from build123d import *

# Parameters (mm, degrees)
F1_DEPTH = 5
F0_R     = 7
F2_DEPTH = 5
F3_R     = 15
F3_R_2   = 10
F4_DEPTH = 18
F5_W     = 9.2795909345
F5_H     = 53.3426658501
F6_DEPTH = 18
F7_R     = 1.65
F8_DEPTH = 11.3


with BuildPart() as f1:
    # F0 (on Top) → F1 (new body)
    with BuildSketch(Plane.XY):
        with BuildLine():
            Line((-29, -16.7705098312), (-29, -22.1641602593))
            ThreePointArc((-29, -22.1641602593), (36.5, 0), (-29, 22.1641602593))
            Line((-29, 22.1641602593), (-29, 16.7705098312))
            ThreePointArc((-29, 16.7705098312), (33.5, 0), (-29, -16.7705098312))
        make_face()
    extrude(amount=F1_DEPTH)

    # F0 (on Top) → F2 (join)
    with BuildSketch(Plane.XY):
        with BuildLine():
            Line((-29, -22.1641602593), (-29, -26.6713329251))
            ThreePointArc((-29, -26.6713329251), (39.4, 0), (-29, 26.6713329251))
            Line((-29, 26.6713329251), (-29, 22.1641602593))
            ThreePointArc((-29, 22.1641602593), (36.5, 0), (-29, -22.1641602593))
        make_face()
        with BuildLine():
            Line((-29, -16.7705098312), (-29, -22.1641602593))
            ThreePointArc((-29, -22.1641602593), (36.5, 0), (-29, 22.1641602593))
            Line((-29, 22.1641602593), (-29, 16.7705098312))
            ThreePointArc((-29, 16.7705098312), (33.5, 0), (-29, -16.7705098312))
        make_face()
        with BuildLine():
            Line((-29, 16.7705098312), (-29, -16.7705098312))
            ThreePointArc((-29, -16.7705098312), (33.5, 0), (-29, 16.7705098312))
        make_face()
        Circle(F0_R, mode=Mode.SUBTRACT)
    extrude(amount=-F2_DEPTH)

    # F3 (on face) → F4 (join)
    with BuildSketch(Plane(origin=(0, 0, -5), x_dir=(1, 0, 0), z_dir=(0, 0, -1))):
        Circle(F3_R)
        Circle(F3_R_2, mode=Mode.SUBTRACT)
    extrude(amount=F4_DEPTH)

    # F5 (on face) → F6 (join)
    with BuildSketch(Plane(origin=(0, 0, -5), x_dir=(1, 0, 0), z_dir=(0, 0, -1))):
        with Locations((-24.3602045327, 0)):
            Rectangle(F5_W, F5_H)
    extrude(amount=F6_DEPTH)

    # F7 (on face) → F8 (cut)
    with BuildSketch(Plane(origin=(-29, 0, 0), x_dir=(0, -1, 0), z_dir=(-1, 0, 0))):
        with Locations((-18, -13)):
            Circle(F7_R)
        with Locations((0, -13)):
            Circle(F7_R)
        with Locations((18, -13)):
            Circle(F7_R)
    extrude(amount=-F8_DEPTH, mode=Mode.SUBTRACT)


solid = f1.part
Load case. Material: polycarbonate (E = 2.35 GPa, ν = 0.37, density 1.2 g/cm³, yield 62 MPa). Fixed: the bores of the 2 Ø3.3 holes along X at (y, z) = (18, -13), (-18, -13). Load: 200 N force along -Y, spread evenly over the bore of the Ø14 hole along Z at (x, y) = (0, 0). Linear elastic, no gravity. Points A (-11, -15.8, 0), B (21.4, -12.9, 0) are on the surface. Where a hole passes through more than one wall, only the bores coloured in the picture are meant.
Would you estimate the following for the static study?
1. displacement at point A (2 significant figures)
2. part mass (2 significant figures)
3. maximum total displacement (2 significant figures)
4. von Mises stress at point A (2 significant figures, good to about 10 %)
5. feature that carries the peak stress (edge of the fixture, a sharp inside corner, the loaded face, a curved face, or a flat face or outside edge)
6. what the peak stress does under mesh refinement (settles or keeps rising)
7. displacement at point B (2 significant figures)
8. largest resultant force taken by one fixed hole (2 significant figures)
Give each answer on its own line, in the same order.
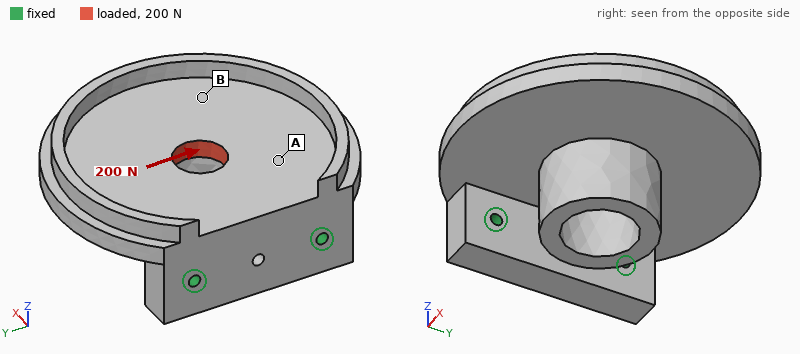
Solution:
0.042 mm
48 g
0.13 mm
1.0 MPa
edge of the fixture
keeps rising
0.099 mm
170 N
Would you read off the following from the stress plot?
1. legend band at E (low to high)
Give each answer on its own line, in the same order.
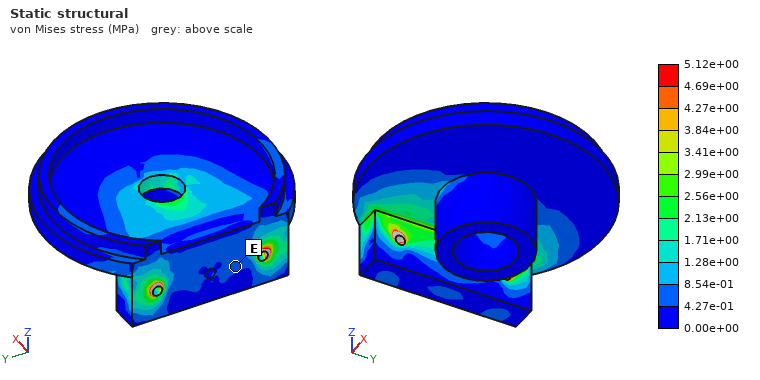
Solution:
4.27e-01 to 8.54e-01 MPa
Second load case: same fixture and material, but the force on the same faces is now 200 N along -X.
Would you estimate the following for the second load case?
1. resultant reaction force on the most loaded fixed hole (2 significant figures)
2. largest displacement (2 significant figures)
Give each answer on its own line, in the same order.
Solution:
100 N
0.17 mm
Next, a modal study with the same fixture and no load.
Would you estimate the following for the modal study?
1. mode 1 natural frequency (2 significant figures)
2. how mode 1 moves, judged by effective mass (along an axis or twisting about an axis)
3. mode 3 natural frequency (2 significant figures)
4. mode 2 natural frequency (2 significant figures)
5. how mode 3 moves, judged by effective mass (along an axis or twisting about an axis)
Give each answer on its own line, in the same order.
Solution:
340 Hz
along Z
1200 Hz
890 Hz
along Y
